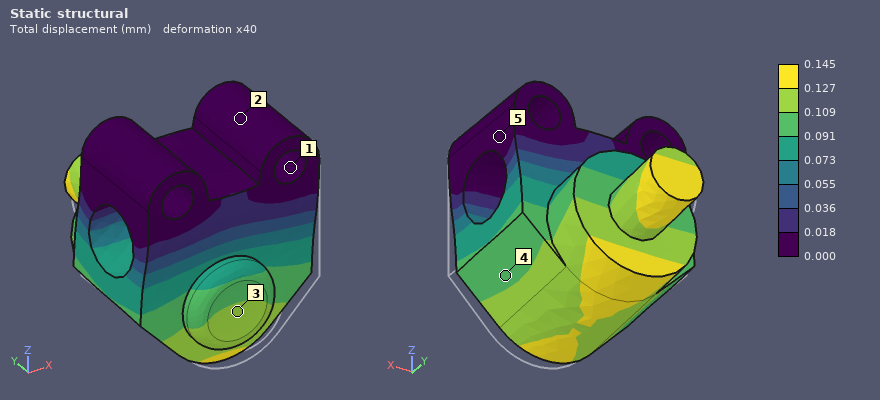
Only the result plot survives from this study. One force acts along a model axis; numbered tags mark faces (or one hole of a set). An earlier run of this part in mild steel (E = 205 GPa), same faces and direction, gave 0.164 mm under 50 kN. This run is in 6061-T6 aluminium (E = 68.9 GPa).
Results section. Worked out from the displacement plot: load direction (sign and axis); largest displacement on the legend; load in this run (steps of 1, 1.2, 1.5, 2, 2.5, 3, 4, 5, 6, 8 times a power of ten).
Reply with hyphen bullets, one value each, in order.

- +Y
- 0.145 mm
- 15 kN
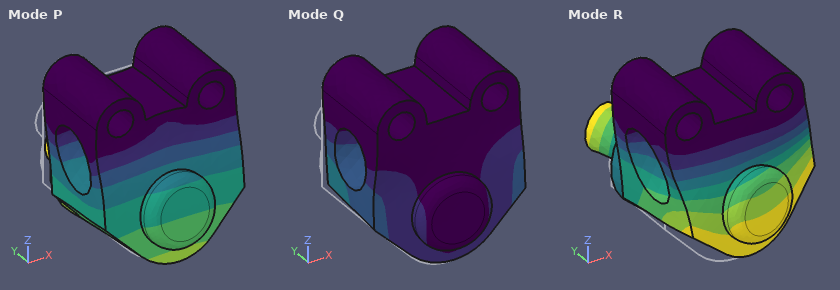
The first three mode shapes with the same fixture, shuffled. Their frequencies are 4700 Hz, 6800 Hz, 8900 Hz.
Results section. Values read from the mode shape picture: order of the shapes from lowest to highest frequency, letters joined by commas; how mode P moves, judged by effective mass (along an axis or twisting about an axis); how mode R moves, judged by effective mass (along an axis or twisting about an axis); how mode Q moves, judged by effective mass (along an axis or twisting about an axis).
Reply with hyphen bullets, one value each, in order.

- P, Q, R
- along Y
- along X
- along X
